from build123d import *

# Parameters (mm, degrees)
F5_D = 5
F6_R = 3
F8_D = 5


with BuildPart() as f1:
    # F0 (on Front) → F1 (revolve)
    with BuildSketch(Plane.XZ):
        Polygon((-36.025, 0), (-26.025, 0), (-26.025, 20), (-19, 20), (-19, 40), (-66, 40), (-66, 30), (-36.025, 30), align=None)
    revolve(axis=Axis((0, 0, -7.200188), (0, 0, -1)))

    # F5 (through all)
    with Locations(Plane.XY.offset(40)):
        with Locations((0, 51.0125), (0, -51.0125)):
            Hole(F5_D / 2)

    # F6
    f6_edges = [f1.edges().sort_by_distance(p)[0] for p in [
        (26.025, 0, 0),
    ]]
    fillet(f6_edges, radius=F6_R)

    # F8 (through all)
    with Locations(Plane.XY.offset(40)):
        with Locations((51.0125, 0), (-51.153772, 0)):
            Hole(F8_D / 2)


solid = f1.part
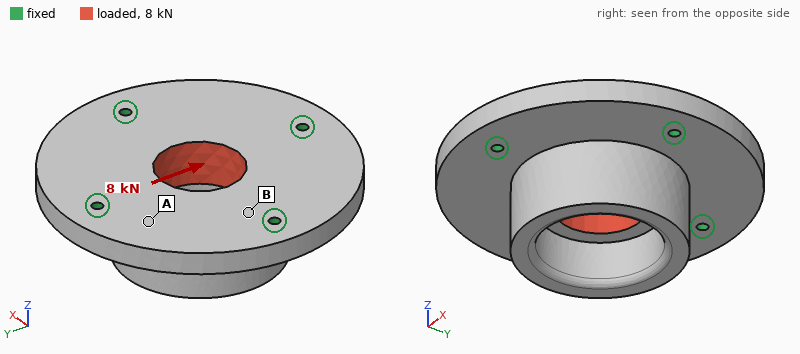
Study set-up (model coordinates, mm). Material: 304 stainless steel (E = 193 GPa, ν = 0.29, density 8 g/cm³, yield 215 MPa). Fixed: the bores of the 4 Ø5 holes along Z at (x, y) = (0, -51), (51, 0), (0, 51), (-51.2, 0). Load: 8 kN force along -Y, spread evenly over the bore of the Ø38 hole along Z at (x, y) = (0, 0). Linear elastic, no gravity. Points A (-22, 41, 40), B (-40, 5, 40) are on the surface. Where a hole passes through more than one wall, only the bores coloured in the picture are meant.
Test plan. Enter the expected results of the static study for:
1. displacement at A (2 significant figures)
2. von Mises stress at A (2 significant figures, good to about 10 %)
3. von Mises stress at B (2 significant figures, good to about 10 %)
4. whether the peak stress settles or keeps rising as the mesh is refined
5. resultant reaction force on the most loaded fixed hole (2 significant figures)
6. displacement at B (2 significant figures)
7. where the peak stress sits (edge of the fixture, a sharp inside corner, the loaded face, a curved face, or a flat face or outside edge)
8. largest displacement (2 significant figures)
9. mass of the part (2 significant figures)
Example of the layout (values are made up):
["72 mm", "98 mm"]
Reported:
["1.1 µm", "1.8 MPa", "3.4 MPa", "keeps rising", "2.4 kN", "0.62 µm", "edge of the fixture", "1.9 µm", "1.5 kg"]
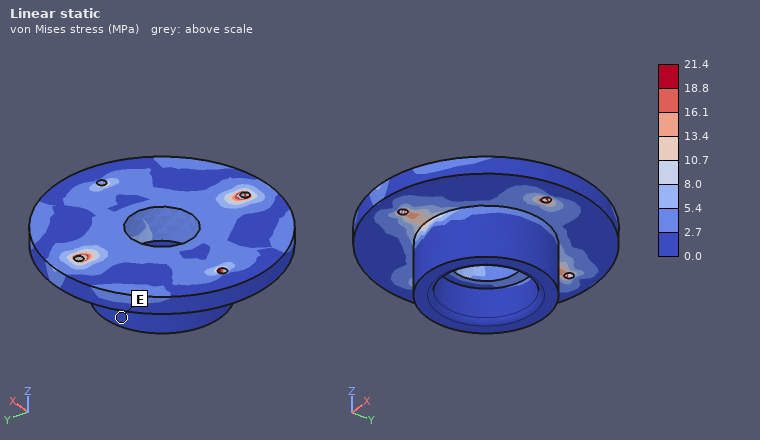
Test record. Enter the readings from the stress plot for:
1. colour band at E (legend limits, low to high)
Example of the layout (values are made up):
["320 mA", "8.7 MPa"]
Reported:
["0.0 to 2.7 MPa"]
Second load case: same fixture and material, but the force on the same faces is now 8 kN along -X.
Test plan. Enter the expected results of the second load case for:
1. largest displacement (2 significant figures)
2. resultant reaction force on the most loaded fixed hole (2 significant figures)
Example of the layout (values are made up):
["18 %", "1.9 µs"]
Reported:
["1.9 µm", "2.4 kN"]
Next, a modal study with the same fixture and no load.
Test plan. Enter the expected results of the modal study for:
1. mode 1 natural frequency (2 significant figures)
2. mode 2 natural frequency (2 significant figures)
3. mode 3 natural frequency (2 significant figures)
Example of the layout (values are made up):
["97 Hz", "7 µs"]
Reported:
["5900 Hz", "6000 Hz", "6000 Hz"]
